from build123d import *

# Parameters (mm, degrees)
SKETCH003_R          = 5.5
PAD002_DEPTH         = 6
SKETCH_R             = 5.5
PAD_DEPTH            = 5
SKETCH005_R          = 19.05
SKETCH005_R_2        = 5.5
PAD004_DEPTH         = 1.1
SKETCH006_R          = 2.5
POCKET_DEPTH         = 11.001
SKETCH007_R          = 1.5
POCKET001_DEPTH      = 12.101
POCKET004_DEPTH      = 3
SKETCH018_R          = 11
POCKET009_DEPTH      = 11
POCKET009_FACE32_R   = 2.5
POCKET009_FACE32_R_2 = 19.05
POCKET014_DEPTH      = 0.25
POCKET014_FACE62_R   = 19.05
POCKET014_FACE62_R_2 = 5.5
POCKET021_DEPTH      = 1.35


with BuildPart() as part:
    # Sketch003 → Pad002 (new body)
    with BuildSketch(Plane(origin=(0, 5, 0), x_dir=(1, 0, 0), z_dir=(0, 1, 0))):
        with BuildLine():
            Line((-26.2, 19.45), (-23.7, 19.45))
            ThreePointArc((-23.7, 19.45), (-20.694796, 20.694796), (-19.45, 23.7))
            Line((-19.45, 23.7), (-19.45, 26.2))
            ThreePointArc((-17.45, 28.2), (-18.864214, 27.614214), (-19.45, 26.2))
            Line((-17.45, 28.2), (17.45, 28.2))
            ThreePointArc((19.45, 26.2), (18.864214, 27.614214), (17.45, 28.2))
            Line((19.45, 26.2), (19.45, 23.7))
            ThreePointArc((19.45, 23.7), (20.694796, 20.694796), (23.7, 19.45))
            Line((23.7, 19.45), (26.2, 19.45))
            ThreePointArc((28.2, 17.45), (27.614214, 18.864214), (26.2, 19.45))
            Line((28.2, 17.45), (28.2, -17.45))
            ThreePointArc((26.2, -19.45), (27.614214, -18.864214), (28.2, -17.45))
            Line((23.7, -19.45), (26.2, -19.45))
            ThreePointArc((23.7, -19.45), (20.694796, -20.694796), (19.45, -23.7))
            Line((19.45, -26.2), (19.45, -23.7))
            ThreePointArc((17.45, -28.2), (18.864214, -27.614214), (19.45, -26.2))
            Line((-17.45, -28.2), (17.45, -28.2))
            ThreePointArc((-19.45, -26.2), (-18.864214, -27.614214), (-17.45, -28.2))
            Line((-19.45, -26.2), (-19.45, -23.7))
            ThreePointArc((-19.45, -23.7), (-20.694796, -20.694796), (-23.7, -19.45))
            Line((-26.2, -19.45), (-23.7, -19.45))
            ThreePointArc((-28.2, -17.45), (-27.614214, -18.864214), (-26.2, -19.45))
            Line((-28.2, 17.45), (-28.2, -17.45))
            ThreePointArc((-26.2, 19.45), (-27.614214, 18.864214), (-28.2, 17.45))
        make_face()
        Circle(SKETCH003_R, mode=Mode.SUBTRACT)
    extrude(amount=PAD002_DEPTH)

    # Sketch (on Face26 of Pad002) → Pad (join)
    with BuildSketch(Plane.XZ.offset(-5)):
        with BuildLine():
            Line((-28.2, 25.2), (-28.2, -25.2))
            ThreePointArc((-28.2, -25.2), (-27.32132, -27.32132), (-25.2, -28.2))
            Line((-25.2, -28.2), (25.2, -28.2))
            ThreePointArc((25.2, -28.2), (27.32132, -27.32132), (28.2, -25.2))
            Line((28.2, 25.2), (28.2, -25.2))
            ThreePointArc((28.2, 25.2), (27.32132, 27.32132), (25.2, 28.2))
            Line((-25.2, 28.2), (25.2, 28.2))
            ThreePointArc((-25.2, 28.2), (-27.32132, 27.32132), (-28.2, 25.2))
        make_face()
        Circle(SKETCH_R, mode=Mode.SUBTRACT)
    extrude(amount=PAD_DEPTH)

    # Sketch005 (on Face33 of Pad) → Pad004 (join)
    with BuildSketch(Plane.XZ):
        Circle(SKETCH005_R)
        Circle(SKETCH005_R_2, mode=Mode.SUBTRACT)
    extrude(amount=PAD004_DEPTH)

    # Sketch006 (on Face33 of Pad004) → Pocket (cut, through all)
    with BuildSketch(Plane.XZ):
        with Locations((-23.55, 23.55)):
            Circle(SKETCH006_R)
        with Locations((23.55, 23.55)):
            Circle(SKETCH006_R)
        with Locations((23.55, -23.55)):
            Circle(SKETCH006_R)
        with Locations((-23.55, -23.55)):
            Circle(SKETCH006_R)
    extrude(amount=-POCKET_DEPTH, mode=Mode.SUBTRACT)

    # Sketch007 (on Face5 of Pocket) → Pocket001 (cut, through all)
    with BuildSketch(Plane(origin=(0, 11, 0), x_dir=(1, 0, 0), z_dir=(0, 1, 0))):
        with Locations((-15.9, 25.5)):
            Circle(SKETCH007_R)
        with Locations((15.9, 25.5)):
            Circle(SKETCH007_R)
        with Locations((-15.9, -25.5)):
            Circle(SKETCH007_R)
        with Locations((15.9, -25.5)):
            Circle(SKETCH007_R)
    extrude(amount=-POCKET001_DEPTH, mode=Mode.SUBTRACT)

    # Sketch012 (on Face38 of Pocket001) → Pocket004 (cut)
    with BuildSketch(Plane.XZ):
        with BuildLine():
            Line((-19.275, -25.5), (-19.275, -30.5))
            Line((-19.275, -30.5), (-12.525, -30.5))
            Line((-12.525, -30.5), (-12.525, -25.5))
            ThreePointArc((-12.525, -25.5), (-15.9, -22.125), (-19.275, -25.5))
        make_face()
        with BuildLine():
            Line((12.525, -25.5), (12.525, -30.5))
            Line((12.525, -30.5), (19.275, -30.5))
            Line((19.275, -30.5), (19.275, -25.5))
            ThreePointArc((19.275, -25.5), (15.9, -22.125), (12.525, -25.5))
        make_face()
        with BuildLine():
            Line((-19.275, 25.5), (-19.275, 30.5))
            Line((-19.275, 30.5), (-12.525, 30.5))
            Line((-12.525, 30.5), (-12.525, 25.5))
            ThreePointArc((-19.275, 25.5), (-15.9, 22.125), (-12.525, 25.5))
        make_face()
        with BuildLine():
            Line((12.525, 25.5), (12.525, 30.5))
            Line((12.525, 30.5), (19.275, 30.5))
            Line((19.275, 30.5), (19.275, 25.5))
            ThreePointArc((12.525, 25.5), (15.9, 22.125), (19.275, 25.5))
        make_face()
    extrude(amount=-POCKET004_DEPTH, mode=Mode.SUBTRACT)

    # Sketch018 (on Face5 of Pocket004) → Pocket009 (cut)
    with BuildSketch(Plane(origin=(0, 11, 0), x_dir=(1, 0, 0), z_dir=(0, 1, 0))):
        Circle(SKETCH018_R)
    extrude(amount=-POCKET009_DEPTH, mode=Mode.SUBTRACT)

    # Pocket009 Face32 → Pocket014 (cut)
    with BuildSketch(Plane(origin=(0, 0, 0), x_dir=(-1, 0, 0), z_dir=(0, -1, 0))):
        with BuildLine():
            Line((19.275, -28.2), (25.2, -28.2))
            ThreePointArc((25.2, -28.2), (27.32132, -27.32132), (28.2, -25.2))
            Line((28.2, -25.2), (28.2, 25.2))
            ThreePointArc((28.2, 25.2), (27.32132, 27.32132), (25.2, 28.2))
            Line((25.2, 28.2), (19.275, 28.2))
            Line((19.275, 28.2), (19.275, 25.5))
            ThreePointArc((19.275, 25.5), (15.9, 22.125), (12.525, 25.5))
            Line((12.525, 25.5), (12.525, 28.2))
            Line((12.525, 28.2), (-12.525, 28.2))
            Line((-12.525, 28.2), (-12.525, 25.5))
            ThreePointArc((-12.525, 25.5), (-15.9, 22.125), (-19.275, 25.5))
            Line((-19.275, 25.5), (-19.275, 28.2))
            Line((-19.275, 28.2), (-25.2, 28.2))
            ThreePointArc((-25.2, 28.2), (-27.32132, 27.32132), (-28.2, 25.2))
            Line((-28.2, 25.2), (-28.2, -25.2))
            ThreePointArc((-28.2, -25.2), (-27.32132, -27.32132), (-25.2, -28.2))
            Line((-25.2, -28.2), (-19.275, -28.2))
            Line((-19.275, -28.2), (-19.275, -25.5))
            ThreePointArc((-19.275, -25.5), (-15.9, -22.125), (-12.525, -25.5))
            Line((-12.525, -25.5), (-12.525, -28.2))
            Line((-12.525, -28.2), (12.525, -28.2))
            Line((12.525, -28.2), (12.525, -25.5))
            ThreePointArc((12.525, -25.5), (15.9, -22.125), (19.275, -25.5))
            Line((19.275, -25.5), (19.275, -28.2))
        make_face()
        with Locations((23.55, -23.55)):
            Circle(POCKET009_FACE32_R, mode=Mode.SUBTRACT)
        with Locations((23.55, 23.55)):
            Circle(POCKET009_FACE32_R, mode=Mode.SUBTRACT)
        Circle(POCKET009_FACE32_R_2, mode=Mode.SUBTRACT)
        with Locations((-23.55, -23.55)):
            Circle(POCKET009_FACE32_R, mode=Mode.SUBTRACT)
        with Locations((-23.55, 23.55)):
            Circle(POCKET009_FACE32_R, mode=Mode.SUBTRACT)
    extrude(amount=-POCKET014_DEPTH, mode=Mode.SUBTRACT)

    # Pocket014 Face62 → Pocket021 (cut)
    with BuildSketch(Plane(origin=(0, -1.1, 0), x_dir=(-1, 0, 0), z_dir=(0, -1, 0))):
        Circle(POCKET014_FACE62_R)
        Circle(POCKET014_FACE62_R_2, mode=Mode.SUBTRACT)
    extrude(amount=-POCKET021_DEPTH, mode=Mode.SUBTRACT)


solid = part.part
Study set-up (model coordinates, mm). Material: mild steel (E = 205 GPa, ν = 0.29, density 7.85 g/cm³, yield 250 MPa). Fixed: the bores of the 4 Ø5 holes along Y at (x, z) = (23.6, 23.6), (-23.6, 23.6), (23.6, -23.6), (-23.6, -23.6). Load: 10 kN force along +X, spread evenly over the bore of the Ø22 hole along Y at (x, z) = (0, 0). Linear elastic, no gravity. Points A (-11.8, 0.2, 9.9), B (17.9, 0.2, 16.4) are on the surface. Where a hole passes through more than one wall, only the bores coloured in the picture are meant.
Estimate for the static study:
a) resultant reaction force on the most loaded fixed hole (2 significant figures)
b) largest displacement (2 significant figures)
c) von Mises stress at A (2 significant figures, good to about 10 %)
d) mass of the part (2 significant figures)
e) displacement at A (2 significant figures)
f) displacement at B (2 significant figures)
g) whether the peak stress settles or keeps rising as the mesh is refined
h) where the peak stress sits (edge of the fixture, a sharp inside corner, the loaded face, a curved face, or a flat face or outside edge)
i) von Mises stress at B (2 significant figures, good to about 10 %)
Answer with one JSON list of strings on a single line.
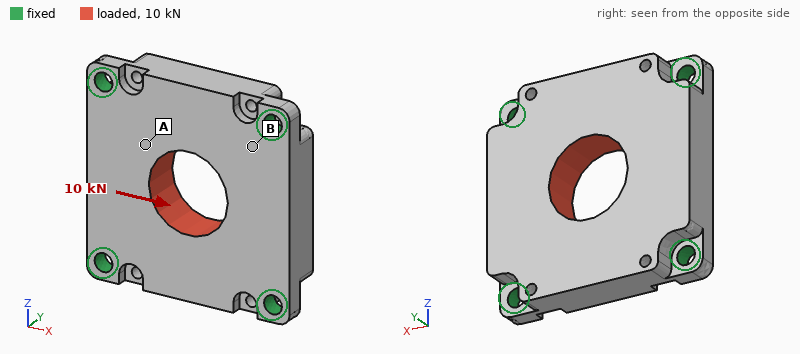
["2.7 kN", "4.9 µm", "15 MPa", "210 g", "3.6 µm", "2.2 µm", "keeps rising", "edge of the fixture", "30 MPa"]
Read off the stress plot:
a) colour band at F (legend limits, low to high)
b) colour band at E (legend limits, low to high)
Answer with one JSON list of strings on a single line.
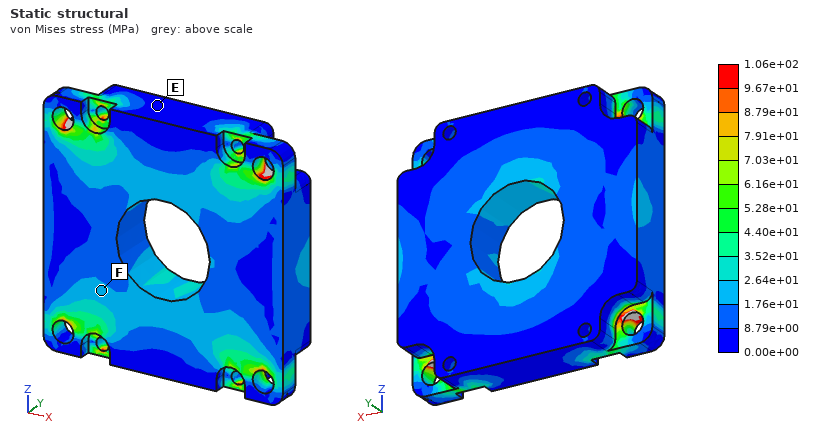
["1.76e+01 to 2.64e+01 MPa", "0.00e+00 to 8.79e+00 MPa"]
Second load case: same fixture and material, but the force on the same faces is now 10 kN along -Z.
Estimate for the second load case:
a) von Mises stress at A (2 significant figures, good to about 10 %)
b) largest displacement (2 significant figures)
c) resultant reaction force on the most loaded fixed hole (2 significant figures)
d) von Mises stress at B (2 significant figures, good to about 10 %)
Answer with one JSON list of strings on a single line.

["16 MPa", "4.4 µm", "2.7 kN", "33 MPa"]
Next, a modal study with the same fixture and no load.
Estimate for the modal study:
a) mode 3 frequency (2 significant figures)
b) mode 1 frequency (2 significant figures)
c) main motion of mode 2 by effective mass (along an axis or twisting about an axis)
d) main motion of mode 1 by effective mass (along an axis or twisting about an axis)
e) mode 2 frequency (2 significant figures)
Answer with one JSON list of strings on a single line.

["17 kHz", "11 kHz", "twisting about X", "along Y", "16 kHz"]
